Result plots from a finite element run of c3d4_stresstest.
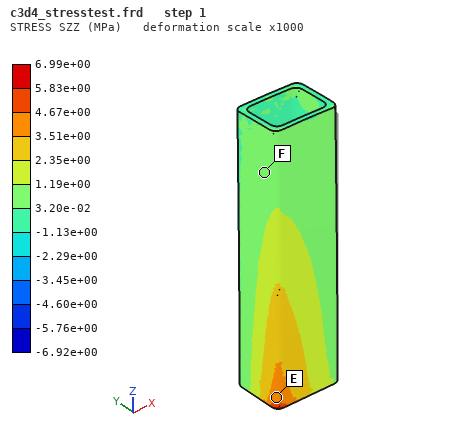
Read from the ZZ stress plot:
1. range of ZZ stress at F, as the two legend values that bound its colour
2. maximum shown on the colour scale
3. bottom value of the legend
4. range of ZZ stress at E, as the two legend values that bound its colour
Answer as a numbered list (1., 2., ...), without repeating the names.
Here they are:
1. 3.20e-02 to 1.19e+00 MPa
2. 6.99e+00 MPa
3. -6.92e+00 MPa
4. 3.51e+00 to 4.67e+00 MPa
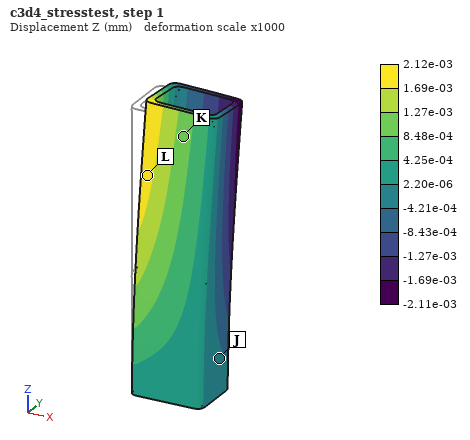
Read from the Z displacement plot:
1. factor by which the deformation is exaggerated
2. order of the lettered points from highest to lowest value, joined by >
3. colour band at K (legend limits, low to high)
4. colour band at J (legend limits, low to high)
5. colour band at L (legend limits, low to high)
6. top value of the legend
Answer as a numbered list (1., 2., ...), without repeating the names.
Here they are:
1. 1000
2. L > K > J
3. 8.48e-04 to 1.27e-03 mm
4. -4.21e-04 to 2.20e-06 mm
5. 1.69e-03 to 2.12e-03 mm
6. 2.12e-03 mm
